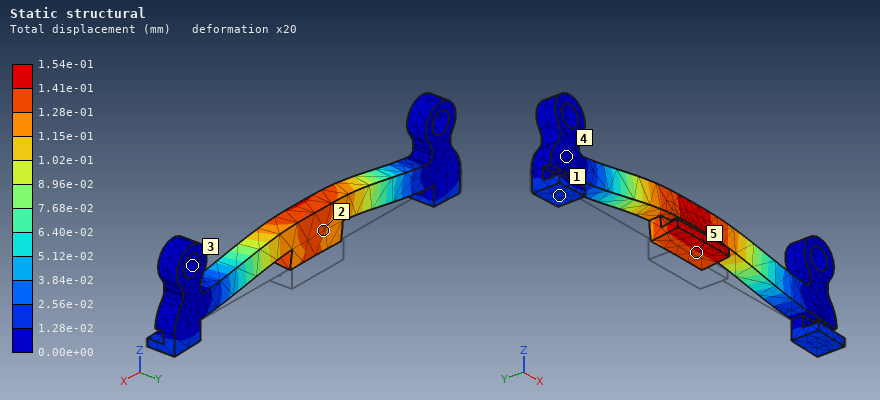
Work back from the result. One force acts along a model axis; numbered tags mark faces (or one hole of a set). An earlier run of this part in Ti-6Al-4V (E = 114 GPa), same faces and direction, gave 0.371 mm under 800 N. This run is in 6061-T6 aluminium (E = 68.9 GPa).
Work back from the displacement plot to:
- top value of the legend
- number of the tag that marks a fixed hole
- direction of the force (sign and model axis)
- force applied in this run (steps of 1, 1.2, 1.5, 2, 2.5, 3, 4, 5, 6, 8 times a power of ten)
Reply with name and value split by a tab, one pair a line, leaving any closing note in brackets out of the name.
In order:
top value of the legend	1.54e-01 mm
number of the tag that marks a fixed hole	3
direction of the force	+Z
force applied in this run	200 N
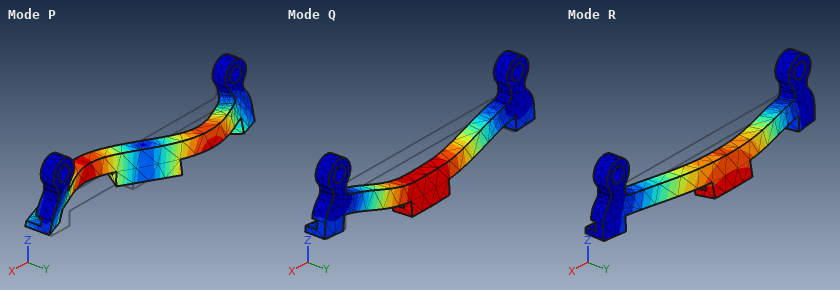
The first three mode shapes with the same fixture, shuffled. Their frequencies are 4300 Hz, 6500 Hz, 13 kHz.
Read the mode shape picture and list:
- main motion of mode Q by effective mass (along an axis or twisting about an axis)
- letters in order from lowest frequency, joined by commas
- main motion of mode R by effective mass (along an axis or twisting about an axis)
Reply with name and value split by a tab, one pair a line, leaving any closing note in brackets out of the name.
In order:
main motion of mode Q by effective mass	along Z
letters in order from lowest frequency, joined by commas	R, Q, P
main motion of mode R by effective mass	along Y
